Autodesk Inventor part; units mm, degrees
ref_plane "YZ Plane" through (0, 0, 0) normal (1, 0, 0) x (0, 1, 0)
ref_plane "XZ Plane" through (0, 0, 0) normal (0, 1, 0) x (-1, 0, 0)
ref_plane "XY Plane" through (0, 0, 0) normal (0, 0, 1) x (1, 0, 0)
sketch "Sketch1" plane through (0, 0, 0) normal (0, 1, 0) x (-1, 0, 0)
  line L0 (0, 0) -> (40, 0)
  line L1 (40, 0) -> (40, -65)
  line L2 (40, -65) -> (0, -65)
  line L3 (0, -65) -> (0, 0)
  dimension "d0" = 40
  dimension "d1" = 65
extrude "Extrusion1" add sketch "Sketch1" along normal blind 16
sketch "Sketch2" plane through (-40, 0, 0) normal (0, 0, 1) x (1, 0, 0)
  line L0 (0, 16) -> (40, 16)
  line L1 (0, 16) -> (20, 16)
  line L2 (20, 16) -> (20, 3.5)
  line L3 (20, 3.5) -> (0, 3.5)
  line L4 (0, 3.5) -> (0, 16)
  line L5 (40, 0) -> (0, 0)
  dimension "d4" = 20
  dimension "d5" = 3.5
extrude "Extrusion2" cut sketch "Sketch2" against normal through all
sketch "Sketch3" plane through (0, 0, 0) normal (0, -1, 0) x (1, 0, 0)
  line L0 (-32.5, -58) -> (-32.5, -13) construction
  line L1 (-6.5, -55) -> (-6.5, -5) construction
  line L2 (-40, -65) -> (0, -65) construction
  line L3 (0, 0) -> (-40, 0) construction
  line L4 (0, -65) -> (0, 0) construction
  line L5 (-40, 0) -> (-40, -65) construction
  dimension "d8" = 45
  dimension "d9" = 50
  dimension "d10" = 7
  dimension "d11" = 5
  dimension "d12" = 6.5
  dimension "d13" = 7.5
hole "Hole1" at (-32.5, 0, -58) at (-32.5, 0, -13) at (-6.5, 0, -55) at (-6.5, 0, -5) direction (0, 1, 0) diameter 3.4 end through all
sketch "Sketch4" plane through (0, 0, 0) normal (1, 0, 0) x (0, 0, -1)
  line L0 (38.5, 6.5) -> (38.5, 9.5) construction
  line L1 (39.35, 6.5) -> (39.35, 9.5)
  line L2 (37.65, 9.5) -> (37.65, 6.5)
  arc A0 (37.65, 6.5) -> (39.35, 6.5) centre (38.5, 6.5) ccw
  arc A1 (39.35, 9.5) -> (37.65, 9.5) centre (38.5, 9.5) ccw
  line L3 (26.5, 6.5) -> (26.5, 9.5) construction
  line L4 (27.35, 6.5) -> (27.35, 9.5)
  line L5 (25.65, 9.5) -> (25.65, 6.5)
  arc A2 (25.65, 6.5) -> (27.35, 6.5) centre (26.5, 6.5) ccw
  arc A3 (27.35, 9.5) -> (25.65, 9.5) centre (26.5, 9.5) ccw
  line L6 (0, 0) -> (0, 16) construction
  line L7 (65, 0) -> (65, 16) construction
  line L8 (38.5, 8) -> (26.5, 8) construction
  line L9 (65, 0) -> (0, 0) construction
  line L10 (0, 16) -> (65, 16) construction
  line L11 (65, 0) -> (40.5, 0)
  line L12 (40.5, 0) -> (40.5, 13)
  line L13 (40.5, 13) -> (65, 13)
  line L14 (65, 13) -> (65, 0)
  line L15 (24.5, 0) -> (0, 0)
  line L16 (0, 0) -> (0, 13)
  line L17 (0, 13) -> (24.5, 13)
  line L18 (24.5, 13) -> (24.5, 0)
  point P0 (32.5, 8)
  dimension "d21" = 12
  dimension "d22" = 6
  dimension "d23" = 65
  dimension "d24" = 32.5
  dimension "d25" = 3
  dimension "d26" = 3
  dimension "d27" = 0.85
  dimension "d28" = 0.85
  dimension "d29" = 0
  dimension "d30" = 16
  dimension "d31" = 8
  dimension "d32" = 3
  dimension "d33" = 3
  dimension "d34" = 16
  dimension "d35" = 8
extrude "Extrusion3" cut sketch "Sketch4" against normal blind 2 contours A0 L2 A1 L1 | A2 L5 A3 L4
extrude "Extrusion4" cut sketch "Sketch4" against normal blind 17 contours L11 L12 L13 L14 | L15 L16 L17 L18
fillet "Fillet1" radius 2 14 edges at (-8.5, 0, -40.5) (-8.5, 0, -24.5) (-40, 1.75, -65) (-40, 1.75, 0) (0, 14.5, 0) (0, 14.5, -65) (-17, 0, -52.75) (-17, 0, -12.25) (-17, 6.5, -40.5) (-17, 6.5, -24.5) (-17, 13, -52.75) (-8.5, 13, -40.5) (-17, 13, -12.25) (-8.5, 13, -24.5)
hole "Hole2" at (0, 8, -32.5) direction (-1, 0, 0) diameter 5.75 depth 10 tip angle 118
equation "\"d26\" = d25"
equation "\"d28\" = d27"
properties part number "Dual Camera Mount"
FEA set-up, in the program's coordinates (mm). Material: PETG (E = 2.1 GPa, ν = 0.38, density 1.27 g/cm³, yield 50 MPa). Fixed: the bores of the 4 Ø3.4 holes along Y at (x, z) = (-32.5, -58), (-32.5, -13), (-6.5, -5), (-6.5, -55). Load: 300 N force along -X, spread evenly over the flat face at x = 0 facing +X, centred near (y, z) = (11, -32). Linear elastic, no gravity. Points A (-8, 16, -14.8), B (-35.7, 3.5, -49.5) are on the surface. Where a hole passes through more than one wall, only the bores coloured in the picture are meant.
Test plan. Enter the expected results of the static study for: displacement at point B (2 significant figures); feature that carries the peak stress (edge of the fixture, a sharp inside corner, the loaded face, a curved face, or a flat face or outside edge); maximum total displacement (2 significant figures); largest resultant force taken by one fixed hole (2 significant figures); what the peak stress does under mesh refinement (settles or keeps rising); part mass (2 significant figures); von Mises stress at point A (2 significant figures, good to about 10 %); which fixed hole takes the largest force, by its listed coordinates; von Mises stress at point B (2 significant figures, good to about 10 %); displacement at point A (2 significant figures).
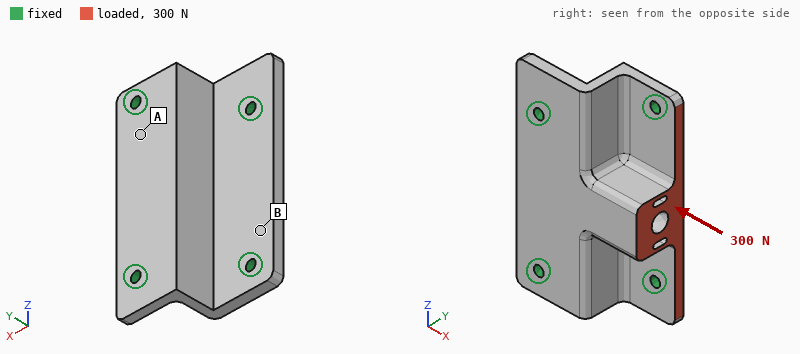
13 µm
edge of the fixture
71 µm
110 N
keeps rising
18 g
2.5 MPa
(-6.5, -55)
0.88 MPa
37 µm
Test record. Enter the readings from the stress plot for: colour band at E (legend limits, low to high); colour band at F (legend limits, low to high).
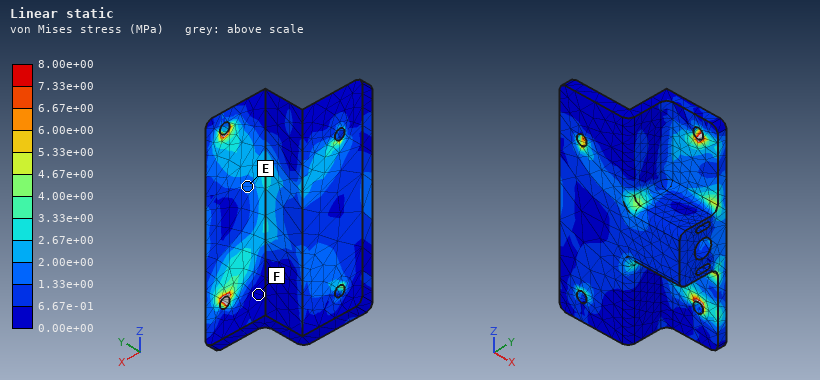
1.33e+00 to 2.00e+00 MPa
0.00e+00 to 6.67e-01 MPa
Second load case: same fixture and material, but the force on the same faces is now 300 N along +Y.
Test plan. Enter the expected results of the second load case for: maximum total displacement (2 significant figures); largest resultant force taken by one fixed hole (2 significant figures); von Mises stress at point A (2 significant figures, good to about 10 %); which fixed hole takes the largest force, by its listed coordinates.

0.46 mm
190 N
10 MPa
(-6.5, -55)
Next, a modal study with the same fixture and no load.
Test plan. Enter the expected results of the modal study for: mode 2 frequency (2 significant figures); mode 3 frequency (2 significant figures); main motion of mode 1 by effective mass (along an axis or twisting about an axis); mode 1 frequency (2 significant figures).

2900 Hz
3500 Hz
along Y
1700 Hz
